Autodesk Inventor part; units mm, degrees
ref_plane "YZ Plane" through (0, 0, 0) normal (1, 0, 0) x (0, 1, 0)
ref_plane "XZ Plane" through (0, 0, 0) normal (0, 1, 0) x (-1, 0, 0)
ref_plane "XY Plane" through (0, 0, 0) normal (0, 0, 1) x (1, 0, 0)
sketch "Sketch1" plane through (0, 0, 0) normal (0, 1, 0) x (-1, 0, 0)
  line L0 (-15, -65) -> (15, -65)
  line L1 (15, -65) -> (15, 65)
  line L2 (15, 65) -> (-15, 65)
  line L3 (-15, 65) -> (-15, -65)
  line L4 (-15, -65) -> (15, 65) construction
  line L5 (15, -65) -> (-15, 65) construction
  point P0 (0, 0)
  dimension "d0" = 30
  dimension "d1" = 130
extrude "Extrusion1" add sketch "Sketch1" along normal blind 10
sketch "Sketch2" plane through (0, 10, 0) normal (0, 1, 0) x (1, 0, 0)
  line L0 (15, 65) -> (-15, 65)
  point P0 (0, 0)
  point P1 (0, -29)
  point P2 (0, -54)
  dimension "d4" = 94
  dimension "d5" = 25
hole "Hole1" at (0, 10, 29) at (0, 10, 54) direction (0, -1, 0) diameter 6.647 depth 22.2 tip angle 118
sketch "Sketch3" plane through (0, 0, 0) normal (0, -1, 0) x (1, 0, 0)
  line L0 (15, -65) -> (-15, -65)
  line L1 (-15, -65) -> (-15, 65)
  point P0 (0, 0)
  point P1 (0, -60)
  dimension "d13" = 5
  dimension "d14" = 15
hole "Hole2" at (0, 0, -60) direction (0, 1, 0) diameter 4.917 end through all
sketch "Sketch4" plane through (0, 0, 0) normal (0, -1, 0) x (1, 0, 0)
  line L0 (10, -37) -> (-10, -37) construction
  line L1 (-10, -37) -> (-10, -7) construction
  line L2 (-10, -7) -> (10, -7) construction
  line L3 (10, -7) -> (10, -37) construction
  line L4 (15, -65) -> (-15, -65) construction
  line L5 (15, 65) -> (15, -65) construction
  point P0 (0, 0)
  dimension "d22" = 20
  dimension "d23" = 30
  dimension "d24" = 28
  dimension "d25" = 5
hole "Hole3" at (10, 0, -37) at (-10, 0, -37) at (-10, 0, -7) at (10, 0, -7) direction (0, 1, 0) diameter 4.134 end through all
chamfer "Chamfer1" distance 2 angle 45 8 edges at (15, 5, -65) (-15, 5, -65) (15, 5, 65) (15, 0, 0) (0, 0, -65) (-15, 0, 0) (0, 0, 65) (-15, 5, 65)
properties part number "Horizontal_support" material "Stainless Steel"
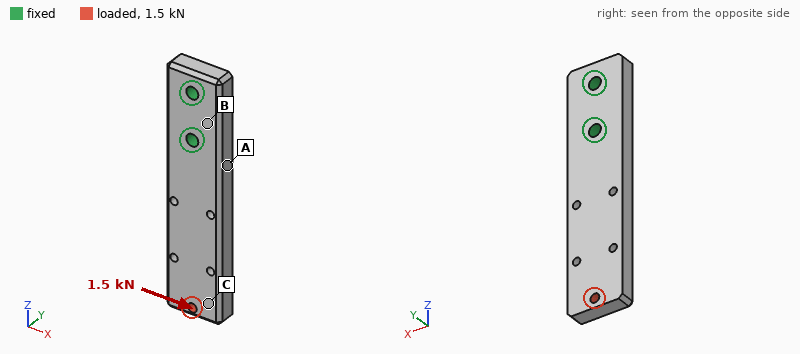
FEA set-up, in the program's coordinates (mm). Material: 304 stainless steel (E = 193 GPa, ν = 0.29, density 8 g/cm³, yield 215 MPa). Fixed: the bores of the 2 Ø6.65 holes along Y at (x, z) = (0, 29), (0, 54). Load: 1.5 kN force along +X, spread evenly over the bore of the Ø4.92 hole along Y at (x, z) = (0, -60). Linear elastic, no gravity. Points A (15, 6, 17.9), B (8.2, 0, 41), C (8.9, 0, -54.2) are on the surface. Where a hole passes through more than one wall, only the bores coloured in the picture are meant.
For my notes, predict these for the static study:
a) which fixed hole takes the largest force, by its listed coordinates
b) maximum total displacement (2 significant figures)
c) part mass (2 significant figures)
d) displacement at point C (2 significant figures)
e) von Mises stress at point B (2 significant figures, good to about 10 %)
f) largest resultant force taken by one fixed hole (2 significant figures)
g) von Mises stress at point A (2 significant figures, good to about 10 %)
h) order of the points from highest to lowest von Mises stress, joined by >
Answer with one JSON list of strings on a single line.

["(0, 29)", "0.14 mm", "300 g", "0.12 mm", "31 MPa", "4.9 kN", "82 MPa", "A > B > C"]
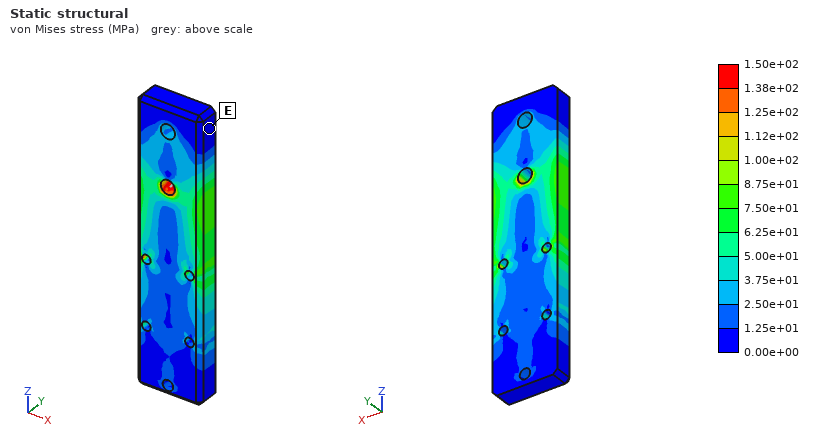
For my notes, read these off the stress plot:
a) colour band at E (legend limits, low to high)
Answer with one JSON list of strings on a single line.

["0.00e+00 to 1.25e+01 MPa"]
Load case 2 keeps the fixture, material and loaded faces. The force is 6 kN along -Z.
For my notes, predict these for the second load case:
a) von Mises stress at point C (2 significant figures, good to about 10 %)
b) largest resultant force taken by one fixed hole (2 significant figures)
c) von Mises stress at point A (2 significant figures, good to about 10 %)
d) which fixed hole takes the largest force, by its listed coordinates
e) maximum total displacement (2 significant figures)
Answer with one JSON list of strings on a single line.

["20 MPa", "5.0 kN", "14 MPa", "(0, 29)", "15 µm"]
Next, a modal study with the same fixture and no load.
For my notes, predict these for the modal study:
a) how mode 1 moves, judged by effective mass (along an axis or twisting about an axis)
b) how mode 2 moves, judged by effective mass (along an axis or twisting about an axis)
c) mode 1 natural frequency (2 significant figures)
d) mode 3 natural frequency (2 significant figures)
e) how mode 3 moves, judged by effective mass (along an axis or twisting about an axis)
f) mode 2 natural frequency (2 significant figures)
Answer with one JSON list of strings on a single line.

["along Y", "along X", "900 Hz", "4700 Hz", "twisting about Z", "2100 Hz"]
